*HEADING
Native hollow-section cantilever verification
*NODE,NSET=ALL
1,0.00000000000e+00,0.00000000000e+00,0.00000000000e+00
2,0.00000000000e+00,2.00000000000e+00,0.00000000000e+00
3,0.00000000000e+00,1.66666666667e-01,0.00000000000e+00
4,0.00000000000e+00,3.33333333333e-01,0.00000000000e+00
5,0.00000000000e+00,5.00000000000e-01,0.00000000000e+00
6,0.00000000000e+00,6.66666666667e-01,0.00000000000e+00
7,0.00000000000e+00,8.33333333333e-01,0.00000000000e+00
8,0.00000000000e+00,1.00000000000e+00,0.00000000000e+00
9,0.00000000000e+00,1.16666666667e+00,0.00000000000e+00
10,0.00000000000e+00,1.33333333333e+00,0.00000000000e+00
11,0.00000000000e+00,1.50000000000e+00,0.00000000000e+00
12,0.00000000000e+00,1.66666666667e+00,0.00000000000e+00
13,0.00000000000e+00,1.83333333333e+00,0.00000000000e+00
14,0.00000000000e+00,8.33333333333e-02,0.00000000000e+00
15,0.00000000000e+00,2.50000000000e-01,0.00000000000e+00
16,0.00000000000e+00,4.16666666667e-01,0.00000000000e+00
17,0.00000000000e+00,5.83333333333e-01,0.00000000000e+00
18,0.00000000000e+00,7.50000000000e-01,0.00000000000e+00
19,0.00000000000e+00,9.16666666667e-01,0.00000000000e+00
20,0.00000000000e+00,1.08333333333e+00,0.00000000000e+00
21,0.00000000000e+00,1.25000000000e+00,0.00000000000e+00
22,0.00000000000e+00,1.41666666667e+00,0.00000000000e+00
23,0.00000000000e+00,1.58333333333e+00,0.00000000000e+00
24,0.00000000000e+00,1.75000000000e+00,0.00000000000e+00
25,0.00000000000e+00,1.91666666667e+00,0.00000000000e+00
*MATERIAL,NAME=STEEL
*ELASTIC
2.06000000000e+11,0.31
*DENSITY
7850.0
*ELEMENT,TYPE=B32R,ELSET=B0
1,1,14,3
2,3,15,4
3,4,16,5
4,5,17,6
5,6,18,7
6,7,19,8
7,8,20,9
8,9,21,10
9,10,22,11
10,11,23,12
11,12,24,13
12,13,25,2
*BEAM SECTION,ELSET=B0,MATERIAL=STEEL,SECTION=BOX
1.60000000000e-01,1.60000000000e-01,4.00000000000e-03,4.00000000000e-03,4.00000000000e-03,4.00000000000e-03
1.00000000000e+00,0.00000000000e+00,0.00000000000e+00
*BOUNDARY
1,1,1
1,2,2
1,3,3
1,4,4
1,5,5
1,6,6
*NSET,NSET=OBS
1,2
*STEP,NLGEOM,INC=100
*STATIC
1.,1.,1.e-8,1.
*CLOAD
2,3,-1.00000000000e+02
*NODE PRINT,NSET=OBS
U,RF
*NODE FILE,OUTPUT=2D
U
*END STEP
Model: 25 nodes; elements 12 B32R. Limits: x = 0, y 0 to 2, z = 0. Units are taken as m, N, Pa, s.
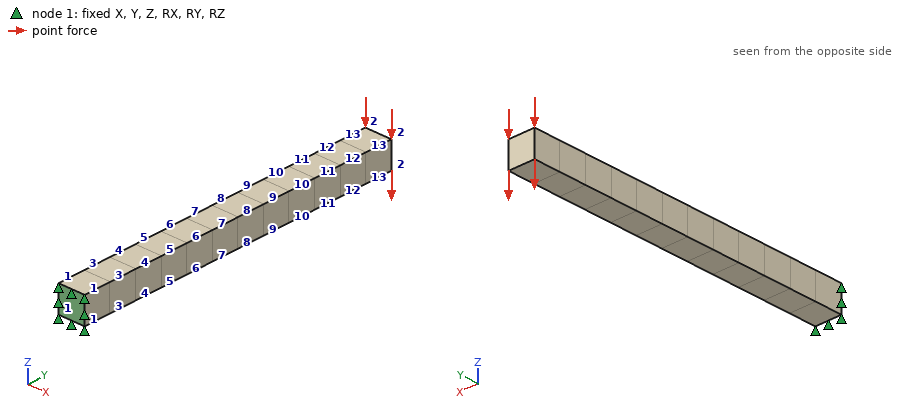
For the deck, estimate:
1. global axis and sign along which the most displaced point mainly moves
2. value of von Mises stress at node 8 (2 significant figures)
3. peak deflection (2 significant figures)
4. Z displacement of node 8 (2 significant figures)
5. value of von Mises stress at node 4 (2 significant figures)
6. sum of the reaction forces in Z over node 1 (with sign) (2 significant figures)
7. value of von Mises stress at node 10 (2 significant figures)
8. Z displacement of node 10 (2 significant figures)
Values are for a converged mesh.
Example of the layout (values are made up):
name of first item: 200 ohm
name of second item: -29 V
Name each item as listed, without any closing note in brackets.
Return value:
global axis and sign along which the most displaced point mainly moves: -Z
value of von Mises stress at node 8: 7.9e+05 Pa
peak deflection: 1.3e-04 m
Z displacement of node 8: -4.0e-05 m
value of von Mises stress at node 4: 1.3e+06 Pa
sum of the reaction forces in Z over node 1 (with sign): 100 N
value of von Mises stress at node 10: 5.3e+05 Pa
Z displacement of node 10: -6.6e-05 m
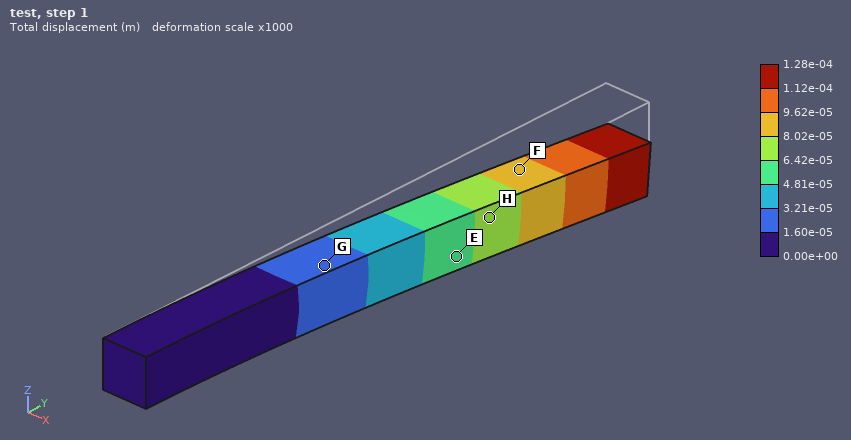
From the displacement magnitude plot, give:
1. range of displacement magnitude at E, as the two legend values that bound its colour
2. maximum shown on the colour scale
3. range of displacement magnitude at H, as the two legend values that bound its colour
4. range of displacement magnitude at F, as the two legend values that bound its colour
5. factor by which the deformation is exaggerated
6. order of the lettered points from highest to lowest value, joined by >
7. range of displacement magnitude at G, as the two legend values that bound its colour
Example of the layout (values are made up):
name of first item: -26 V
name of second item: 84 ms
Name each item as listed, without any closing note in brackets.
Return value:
range of displacement magnitude at E, as the two legend values that bound its colour: 4.81e-05 to 6.42e-05 m
maximum shown on the colour scale: 1.28e-04 m
range of displacement magnitude at H, as the two legend values that bound its colour: 6.42e-05 to 8.02e-05 m
range of displacement magnitude at F, as the two legend values that bound its colour: 8.02e-05 to 9.62e-05 m
factor by which the deformation is exaggerated: 1000
order of the lettered points from highest to lowest value, joined by >: F > H > E > G
range of displacement magnitude at G, as the two legend values that bound its colour: 1.60e-05 to 3.21e-05 m
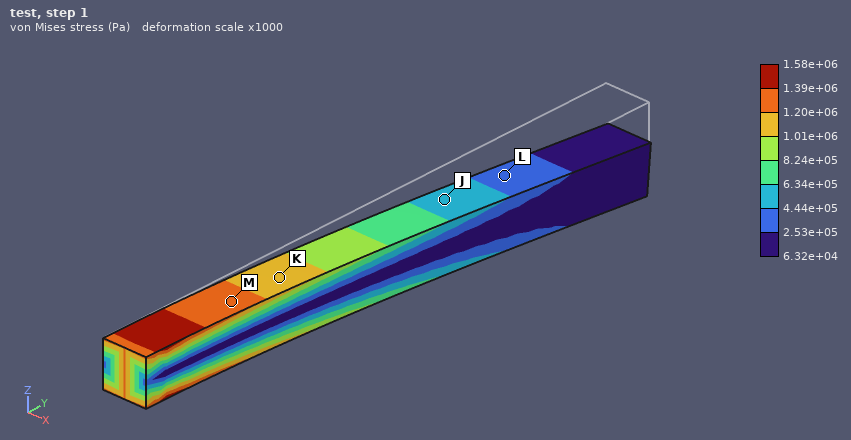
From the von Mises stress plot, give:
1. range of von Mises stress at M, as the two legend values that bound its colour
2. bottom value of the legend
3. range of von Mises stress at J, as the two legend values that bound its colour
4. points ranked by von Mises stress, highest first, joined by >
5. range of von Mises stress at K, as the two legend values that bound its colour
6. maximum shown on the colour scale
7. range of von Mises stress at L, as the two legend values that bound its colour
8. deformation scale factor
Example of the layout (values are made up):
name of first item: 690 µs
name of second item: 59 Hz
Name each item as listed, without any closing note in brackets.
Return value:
range of von Mises stress at M, as the two legend values that bound its colour: 1.20e+06 to 1.39e+06 Pa
bottom value of the legend: 6.32e+04 Pa
range of von Mises stress at J, as the two legend values that bound its colour: 4.44e+05 to 6.34e+05 Pa
points ranked by von Mises stress, highest first, joined by >: M > K > J > L
range of von Mises stress at K, as the two legend values that bound its colour: 1.01e+06 to 1.20e+06 Pa
maximum shown on the colour scale: 1.58e+06 Pa
range of von Mises stress at L, as the two legend values that bound its colour: 2.53e+05 to 4.44e+05 Pa
deformation scale factor: 1000
